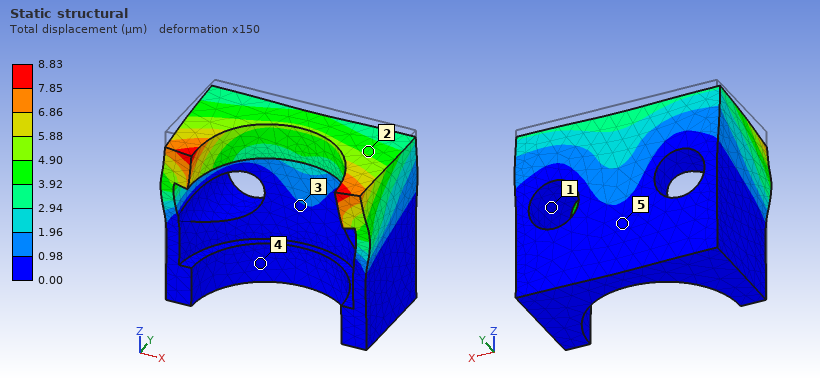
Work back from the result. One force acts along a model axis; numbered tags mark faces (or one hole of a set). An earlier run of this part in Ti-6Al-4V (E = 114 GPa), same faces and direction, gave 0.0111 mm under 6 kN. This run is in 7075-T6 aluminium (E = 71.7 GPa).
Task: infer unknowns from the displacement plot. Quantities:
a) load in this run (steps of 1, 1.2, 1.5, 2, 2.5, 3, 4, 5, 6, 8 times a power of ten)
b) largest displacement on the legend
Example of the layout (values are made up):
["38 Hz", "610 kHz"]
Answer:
["3 kN", "8.83 µm"]
